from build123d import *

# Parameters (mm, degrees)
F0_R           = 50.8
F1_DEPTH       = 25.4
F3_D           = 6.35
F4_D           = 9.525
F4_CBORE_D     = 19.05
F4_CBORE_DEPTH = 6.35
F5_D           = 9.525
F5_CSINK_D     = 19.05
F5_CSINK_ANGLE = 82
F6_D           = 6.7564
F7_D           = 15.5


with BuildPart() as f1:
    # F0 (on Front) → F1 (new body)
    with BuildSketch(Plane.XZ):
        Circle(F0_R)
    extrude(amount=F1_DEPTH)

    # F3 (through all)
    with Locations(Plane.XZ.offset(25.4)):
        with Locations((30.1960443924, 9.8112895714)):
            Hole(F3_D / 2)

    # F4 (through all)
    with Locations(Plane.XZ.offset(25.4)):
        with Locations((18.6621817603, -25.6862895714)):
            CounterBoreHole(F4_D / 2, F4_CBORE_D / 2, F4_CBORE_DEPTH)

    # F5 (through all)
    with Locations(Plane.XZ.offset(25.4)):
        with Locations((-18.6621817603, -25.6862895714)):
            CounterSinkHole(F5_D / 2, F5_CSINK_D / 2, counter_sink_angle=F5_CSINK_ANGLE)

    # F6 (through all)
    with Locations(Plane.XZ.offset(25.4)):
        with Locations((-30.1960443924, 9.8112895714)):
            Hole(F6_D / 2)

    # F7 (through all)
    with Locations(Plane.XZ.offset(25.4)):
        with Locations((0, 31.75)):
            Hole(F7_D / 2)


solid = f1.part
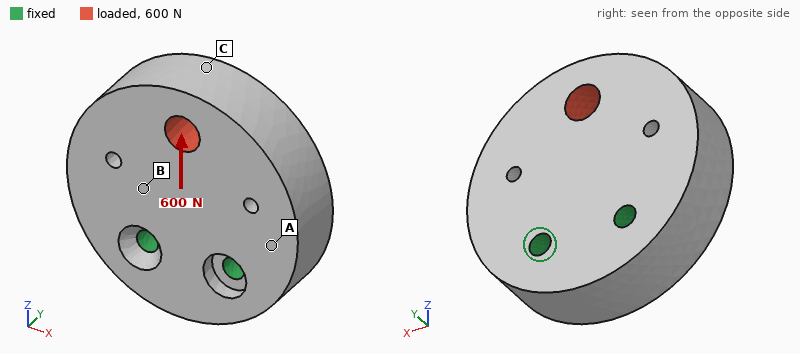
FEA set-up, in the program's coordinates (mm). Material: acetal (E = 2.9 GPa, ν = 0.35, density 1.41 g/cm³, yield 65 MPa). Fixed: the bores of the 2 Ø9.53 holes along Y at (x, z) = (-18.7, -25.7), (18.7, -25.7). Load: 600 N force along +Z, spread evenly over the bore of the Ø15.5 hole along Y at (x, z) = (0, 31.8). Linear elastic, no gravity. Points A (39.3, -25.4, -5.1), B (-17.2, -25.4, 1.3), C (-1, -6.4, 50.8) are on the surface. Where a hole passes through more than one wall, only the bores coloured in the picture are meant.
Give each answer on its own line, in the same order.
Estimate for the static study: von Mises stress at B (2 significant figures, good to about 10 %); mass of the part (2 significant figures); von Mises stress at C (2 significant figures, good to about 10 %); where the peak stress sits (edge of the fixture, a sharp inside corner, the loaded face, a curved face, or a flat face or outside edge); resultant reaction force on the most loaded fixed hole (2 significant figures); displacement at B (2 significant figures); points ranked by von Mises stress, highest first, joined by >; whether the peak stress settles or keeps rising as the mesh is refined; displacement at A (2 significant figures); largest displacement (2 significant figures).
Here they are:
0.42 MPa
270 g
0.68 MPa
edge of the fixture
310 N
5.9 µm
C > B > A
keeps rising
5.8 µm
16 µm
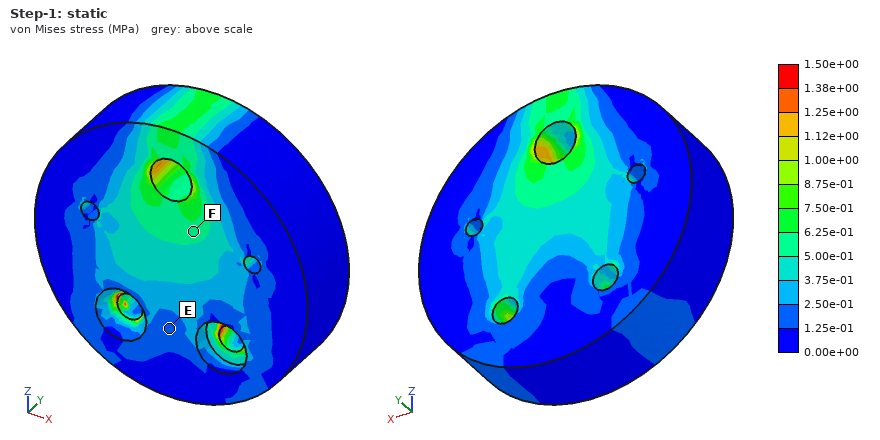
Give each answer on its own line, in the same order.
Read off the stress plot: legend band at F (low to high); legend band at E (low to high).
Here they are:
5.00e-01 to 6.25e-01 MPa
1.25e-01 to 2.50e-01 MPa
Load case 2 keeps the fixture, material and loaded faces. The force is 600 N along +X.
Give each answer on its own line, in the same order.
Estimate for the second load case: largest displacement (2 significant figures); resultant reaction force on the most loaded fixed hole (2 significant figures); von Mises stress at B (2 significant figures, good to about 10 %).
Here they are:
56 µm
830 N
0.63 MPa
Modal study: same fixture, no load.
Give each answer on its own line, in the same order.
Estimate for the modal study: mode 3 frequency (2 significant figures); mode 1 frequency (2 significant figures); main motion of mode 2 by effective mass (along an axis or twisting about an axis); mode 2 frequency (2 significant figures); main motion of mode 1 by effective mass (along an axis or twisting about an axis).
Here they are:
1700 Hz
900 Hz
along X
1600 Hz
along Y
